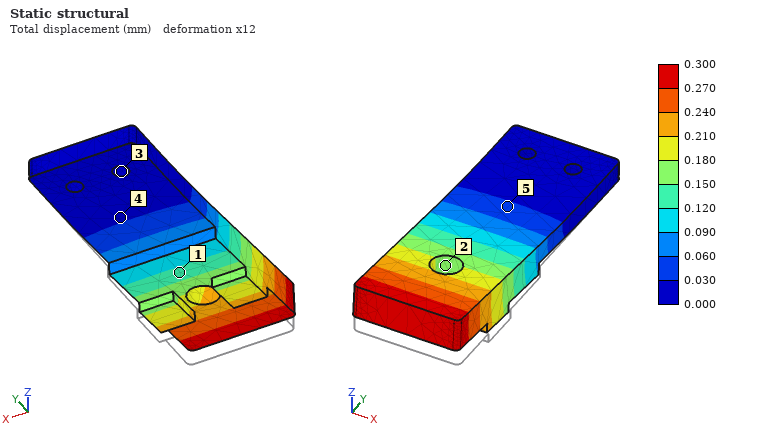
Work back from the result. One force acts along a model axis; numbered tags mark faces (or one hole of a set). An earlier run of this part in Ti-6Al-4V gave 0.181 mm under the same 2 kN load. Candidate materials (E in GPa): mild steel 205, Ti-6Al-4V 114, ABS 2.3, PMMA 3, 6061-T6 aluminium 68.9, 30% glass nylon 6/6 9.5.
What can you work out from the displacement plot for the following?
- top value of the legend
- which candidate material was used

0.300 mm
6061-T6 aluminium
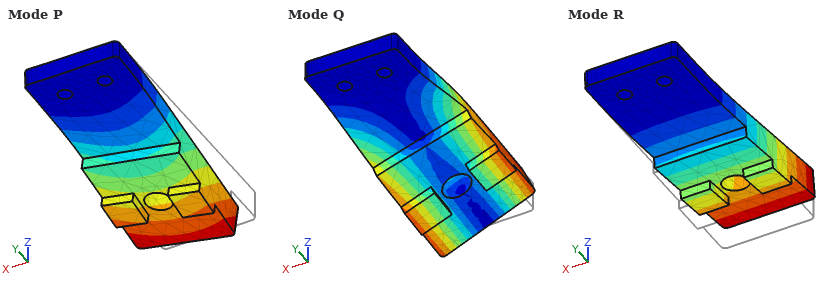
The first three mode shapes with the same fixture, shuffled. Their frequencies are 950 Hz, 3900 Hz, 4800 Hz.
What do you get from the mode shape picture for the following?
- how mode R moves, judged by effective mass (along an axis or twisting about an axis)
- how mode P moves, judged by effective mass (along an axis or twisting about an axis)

along Z
along X
